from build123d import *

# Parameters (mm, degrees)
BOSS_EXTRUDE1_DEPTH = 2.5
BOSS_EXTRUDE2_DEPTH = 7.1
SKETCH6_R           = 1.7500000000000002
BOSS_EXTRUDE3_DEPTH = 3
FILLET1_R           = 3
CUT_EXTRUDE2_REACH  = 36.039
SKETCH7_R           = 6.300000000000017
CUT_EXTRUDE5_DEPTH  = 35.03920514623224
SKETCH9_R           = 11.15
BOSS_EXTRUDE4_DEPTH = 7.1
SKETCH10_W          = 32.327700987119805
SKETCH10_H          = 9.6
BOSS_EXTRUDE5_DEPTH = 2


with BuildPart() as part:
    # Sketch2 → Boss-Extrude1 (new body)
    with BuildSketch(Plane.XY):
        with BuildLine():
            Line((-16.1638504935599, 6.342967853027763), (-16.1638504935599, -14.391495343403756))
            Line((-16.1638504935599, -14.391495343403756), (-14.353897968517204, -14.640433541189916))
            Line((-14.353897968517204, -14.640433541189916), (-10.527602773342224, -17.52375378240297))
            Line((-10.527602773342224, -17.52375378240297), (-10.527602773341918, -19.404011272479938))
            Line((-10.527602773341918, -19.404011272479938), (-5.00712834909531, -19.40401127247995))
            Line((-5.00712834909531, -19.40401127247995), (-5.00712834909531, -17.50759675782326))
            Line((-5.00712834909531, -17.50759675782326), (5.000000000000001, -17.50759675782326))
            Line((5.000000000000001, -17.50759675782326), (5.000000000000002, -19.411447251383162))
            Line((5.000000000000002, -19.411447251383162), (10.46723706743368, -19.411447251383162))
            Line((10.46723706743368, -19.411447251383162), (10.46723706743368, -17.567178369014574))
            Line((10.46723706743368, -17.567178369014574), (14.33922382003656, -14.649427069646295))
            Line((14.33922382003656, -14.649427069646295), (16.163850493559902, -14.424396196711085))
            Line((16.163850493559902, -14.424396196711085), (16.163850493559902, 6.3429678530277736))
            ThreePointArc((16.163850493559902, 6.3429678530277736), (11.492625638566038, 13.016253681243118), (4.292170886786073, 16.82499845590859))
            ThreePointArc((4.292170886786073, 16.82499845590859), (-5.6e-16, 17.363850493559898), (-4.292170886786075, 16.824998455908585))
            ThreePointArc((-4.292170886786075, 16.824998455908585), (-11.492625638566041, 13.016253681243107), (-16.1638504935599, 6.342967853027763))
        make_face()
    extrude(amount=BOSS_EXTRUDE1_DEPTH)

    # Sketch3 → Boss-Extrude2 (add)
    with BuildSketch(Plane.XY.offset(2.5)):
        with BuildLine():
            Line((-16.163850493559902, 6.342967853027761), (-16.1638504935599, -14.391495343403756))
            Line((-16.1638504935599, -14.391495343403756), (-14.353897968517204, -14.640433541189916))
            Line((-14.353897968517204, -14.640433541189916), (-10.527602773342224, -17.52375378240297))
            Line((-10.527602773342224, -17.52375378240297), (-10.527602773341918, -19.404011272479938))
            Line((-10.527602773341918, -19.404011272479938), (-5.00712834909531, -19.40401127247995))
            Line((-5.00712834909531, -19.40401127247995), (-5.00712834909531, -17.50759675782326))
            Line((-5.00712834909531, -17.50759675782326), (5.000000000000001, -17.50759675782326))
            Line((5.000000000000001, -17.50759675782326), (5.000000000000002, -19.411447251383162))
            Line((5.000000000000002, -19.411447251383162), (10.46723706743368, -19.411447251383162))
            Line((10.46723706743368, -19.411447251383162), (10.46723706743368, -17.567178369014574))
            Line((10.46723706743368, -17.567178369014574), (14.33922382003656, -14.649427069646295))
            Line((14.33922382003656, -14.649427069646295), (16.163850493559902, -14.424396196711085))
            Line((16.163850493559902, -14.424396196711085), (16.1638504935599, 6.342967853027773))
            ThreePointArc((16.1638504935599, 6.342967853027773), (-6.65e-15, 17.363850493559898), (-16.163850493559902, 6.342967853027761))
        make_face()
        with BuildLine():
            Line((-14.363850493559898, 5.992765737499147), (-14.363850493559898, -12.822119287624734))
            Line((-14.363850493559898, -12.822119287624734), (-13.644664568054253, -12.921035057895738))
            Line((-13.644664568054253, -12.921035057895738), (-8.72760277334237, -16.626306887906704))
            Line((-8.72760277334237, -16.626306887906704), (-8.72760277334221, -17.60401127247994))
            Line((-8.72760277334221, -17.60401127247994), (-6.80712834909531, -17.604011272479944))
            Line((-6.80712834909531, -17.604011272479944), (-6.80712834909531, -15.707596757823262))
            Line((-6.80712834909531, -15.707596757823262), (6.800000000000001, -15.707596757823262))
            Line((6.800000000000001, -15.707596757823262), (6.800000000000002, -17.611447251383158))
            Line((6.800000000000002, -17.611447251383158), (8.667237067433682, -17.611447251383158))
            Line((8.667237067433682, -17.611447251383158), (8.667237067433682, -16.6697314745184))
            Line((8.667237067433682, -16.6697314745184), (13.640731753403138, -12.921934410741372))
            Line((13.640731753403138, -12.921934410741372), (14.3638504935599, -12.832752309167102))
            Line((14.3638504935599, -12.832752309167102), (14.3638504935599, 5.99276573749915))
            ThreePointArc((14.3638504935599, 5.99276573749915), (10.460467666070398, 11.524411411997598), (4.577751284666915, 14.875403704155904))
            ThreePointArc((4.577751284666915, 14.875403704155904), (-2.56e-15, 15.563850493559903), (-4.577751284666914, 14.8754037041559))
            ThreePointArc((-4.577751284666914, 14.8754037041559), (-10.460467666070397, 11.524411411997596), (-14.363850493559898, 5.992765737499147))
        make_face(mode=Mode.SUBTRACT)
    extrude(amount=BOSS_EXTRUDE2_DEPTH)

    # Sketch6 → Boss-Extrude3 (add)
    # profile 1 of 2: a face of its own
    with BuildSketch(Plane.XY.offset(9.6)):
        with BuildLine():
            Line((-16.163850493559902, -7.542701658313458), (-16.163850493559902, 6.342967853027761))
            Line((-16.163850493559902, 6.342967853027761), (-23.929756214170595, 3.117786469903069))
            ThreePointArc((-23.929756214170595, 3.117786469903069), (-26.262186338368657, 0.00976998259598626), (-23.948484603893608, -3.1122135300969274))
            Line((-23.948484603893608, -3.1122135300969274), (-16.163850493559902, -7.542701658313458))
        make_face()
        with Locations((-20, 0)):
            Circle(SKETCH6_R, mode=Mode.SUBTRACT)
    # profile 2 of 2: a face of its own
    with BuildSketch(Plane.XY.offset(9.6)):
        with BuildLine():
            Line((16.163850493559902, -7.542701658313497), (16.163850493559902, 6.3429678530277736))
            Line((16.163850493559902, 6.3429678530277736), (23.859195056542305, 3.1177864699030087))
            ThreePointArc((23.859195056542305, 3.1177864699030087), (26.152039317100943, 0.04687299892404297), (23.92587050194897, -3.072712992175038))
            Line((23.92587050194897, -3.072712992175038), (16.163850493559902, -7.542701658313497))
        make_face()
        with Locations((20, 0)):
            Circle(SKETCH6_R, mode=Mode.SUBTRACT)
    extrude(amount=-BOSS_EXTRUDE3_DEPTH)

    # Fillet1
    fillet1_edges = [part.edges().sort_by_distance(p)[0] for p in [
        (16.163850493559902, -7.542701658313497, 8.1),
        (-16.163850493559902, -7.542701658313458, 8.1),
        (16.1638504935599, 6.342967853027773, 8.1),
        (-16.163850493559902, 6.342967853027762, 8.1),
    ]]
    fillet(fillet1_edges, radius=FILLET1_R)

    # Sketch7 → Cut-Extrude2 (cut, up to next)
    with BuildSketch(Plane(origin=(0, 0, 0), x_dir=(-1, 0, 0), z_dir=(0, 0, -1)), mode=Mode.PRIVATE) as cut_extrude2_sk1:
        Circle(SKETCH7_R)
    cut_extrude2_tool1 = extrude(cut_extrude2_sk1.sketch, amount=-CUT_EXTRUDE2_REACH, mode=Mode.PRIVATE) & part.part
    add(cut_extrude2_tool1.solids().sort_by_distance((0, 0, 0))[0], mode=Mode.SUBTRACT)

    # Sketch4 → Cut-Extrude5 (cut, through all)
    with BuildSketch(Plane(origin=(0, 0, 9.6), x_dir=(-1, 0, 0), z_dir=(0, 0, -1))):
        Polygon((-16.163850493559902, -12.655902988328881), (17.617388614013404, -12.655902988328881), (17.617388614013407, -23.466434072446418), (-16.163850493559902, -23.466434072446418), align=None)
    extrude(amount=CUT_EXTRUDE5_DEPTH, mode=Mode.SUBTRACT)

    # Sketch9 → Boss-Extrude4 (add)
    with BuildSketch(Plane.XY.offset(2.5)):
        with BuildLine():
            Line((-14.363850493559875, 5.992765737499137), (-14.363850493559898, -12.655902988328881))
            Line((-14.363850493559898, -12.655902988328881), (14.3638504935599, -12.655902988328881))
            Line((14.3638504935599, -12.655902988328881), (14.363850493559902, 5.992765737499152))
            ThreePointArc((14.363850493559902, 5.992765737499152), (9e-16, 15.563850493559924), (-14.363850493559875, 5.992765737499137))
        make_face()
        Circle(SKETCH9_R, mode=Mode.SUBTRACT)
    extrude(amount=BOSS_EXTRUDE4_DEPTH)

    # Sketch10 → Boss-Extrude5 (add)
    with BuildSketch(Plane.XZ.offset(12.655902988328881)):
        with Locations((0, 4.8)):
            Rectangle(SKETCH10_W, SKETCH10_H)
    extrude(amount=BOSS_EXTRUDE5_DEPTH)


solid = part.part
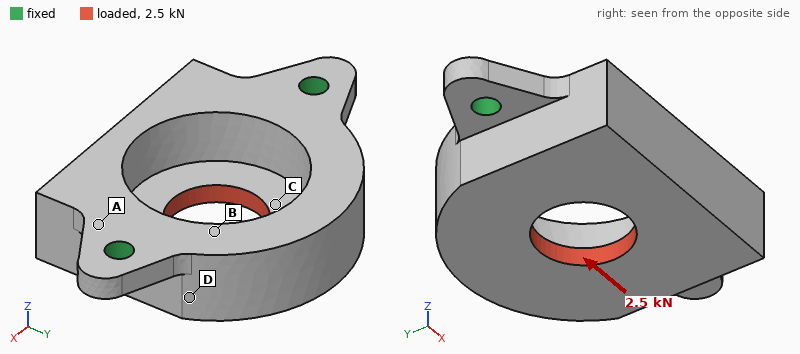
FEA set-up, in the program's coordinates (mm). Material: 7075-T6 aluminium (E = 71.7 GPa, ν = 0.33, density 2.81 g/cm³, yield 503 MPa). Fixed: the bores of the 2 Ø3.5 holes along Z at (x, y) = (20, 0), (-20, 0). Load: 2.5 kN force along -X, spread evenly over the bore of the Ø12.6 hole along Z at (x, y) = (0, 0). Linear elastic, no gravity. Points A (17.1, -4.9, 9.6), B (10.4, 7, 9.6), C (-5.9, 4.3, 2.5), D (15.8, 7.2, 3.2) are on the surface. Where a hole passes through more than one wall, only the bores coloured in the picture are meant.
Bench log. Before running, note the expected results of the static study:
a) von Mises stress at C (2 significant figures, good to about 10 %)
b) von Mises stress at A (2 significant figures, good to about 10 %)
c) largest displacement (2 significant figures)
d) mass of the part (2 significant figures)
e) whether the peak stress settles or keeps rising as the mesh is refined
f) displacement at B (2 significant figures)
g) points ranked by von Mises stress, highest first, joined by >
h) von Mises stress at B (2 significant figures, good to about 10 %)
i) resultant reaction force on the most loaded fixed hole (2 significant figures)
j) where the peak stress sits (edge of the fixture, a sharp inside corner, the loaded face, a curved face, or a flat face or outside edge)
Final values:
40 MPa
19 MPa
15 µm
18 g
keeps rising
4.2 µm
C > B > A > D
30 MPa
1.3 kN
edge of the fixture
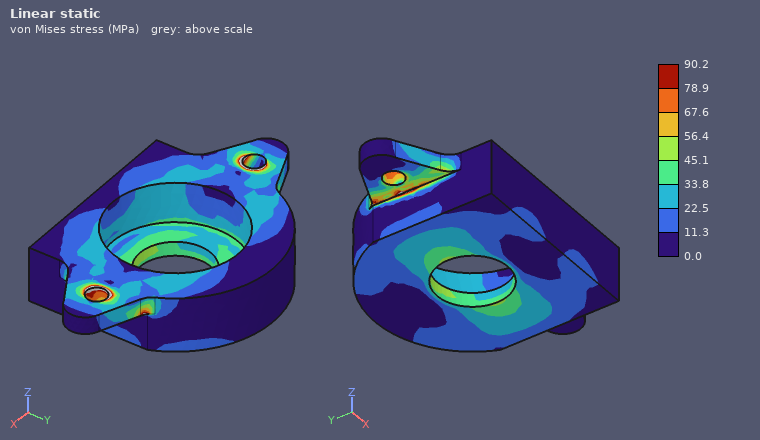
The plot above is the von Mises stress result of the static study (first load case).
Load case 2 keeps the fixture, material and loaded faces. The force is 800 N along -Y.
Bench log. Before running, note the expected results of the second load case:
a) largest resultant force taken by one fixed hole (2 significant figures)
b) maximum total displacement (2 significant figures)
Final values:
400 N
69 µm
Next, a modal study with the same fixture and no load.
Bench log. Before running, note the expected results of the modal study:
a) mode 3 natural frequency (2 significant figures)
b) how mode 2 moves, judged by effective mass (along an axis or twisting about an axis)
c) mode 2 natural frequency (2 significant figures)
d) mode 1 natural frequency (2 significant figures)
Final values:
18 kHz
along Z
12 kHz
4500 Hz
